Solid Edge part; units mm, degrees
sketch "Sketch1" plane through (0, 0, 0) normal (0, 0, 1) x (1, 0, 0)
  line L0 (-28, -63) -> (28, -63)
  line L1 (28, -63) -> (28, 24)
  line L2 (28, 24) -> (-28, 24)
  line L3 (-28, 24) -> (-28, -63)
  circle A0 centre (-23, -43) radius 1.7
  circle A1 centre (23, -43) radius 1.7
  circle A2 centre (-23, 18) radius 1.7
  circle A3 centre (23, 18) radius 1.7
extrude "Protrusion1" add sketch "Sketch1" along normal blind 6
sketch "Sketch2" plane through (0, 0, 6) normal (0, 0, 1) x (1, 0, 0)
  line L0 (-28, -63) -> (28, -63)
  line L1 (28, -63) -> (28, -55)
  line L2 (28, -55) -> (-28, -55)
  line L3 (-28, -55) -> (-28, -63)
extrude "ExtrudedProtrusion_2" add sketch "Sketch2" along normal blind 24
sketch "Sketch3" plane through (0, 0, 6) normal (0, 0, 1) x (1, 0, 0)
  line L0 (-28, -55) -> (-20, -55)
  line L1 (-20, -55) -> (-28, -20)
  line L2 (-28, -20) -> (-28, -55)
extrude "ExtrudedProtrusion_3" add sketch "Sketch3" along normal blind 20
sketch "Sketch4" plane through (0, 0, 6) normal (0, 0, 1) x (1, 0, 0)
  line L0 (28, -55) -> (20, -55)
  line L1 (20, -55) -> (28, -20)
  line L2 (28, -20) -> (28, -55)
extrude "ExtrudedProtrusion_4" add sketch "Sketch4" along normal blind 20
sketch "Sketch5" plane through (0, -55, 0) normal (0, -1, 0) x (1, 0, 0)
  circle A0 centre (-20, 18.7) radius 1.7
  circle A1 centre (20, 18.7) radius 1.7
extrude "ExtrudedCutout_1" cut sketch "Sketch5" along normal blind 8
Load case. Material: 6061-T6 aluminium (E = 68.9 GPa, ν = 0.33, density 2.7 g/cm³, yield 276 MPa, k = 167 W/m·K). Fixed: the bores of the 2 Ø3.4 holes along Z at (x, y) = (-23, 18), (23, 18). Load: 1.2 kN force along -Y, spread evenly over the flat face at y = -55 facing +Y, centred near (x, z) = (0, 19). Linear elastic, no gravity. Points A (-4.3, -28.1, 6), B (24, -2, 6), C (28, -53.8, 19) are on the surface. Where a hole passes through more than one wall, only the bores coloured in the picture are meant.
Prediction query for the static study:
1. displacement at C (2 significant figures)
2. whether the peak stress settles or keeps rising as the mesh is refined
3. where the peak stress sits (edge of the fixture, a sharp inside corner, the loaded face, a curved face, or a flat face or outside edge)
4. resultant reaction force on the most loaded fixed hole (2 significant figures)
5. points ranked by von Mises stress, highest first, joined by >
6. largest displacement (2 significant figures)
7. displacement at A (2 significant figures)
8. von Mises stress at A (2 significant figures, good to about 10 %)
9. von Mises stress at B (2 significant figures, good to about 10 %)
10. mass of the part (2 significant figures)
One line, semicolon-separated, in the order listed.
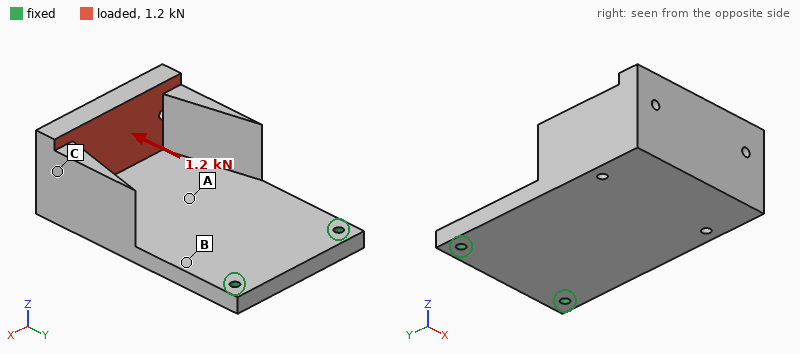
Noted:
0.82 mm; keeps rising; edge of the fixture; 620 N; B > A > C; 1.0 mm; 0.39 mm; 41 MPa; 66 MPa; 120 g
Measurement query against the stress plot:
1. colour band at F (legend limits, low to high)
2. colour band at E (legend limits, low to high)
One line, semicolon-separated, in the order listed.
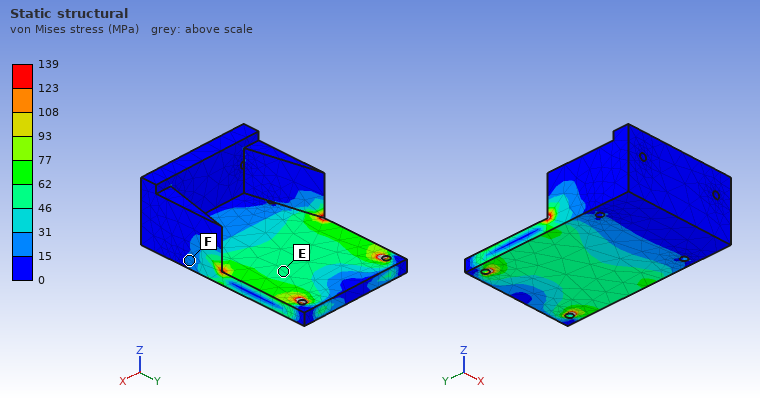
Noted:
15 to 31 MPa; 46 to 62 MPa
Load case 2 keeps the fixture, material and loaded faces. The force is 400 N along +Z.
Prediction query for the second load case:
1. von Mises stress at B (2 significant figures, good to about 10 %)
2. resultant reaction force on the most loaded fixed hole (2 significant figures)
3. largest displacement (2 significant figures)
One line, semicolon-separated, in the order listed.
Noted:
68 MPa; 200 N; 1.2 mm
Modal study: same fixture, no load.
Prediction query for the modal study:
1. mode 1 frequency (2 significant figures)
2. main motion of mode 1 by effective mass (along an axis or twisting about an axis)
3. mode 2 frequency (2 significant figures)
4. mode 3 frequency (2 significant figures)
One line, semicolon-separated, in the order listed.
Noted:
390 Hz; along Z; 1400 Hz; 2900 Hz
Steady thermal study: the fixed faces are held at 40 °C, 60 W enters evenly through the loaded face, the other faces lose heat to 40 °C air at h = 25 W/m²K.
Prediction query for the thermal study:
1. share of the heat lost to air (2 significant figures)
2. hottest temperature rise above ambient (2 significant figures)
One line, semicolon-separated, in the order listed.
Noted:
29 %; 71 K
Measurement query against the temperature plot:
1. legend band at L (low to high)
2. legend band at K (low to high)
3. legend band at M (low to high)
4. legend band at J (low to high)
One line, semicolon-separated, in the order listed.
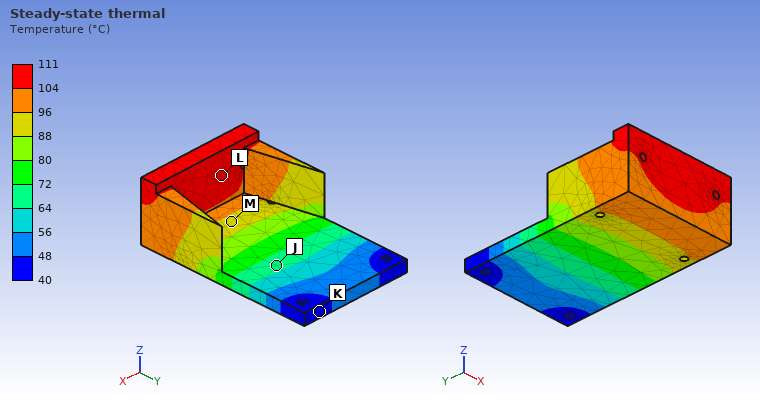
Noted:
104 to 111 °C; 40 to 48 °C; 88 to 96 °C; 64 to 72 °C
